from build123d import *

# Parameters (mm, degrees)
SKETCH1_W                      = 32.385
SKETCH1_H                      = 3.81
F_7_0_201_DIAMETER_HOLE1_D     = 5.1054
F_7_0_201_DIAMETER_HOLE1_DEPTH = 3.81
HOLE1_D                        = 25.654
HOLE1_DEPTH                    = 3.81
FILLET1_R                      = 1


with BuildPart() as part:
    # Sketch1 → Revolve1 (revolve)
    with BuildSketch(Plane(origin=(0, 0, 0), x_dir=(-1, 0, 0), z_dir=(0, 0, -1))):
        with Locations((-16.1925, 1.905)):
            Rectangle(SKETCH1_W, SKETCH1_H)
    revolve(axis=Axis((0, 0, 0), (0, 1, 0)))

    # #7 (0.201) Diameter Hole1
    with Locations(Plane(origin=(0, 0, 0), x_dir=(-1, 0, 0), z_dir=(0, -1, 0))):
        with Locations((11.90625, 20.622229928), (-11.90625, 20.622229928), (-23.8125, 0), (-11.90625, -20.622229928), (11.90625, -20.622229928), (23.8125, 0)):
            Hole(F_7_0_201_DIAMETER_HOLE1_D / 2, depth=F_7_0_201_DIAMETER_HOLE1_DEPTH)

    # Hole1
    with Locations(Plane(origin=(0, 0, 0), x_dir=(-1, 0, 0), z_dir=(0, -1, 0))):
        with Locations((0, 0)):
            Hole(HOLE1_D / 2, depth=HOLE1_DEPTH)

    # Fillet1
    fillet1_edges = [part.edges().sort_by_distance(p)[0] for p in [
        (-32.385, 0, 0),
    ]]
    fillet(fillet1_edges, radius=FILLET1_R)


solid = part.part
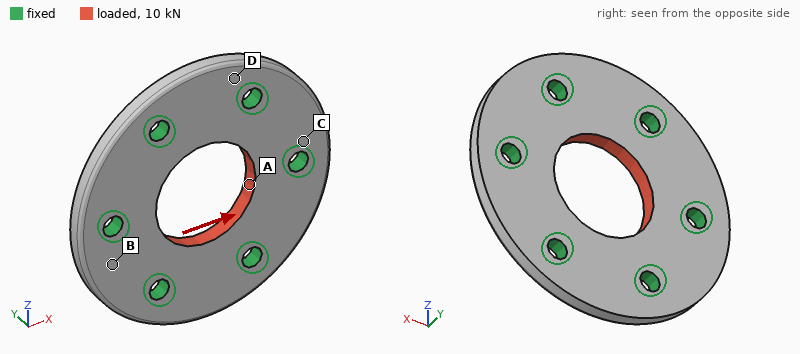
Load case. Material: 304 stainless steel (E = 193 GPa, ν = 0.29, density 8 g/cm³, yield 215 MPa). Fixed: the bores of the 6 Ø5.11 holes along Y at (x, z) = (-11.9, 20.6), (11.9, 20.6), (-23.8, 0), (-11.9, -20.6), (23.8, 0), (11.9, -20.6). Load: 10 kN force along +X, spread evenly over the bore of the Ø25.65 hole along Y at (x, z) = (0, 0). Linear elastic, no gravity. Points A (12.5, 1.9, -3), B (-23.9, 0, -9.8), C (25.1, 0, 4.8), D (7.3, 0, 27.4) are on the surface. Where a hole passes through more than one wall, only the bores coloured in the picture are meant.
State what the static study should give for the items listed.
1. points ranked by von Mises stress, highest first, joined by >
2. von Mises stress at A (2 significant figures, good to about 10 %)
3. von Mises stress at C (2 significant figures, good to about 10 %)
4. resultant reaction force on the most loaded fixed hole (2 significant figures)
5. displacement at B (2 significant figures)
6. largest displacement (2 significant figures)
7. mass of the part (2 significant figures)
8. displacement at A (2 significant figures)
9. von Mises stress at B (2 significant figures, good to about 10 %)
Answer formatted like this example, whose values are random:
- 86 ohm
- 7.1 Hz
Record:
- A > C > B > D
- 34 MPa
- 24 MPa
- 2.3 kN
- 1.2 µm
- 2.7 µm
- 81 g
- 2.2 µm
- 12 MPa
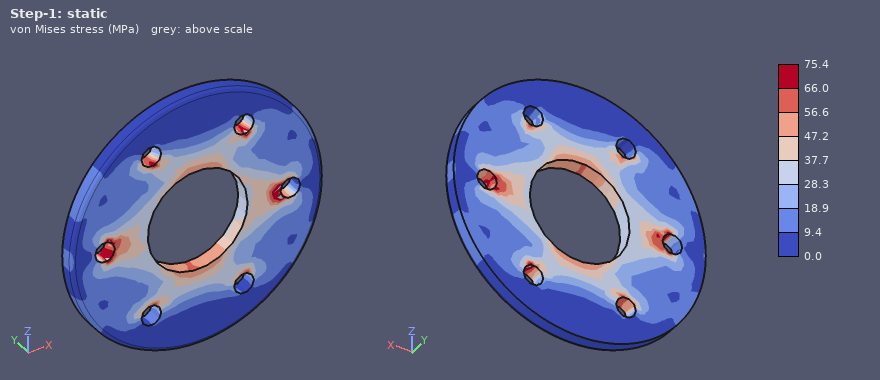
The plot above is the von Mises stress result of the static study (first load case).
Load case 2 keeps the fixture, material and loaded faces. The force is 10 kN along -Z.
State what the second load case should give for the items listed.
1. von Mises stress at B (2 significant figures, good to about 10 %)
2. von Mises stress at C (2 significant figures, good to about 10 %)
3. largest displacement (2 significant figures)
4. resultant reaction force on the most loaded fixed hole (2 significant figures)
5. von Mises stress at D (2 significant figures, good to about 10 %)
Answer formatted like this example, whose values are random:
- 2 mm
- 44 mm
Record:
- 7.3 MPa
- 11 MPa
- 2.8 µm
- 2.0 kN
- 15 MPa
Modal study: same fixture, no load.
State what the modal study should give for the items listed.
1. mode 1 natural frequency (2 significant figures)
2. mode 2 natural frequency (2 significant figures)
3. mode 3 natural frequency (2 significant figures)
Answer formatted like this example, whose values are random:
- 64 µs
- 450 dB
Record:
- 22 kHz
- 23 kHz
- 23 kHz
